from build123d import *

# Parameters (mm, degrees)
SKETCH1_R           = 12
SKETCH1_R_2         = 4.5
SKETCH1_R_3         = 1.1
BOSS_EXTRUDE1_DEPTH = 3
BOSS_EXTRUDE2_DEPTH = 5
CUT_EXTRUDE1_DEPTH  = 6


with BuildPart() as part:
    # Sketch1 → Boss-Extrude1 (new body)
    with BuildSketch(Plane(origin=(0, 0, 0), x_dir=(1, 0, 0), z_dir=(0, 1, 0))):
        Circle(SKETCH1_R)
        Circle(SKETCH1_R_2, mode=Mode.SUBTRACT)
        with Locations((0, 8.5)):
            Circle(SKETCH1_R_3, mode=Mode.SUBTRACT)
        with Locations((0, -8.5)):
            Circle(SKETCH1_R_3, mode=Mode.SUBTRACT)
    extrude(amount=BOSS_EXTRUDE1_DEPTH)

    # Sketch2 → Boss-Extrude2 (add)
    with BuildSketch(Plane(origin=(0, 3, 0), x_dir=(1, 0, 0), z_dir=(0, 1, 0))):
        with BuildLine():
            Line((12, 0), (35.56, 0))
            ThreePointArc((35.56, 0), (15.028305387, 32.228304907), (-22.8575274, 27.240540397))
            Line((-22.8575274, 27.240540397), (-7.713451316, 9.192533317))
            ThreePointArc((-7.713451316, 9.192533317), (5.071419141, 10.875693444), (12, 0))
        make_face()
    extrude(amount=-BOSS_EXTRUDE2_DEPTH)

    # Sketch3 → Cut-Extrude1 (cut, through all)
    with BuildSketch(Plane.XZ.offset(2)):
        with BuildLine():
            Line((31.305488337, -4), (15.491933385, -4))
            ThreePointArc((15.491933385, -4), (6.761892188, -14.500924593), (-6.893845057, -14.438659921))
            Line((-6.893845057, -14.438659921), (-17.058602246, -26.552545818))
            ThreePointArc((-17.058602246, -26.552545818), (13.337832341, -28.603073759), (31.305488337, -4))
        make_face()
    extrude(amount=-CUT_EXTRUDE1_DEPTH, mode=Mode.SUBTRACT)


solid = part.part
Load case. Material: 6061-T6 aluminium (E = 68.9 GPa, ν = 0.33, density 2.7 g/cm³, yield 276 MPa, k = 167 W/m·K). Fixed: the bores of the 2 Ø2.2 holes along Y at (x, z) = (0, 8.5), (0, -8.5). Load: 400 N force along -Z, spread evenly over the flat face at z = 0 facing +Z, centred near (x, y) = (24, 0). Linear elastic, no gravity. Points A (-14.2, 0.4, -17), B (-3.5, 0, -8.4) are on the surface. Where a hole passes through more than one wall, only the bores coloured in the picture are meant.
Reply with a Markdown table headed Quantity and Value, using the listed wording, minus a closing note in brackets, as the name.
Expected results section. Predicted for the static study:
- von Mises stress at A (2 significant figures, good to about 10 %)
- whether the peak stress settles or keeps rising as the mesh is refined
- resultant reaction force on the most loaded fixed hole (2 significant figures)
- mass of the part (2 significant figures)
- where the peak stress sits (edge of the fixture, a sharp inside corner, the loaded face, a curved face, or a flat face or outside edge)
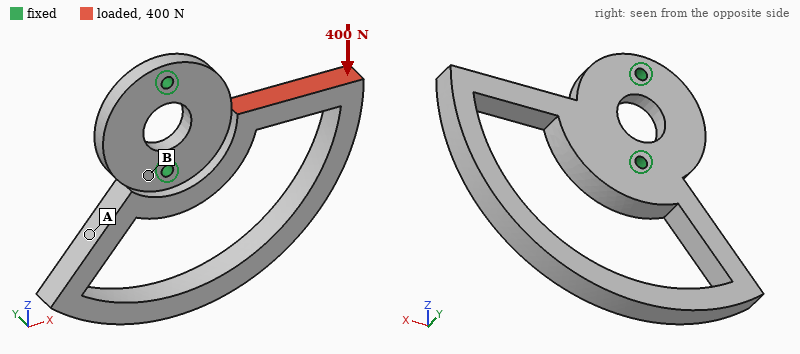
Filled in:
| Quantity | Value |
|---|---|
| von Mises stress at A | 39 MPa |
| whether the peak stress settles or keeps rising as the mesh is refined | keeps rising |
| resultant reaction force on the most loaded fixed hole | 570 N |
| mass of the part | 11 g |
| where the peak stress sits | a sharp inside corner |
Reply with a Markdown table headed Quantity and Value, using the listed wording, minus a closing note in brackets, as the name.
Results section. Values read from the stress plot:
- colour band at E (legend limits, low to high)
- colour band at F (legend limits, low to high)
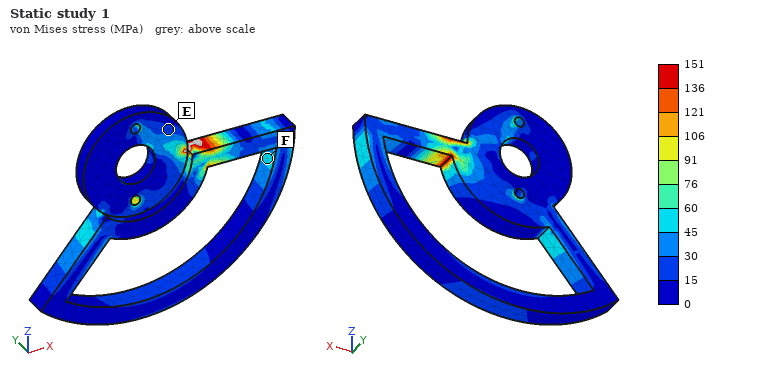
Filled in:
| Quantity | Value |
|---|---|
| colour band at E | 15 to 30 MPa |
| colour band at F | 45 to 60 MPa |
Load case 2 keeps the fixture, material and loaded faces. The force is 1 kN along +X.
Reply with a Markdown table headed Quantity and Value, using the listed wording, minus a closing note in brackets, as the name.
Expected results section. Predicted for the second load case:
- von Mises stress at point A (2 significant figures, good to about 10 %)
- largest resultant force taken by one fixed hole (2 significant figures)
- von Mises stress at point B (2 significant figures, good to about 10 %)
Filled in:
| Quantity | Value |
|---|---|
| von Mises stress at point A | 26 MPa |
| largest resultant force taken by one fixed hole | 580 N |
| von Mises stress at point B | 19 MPa |
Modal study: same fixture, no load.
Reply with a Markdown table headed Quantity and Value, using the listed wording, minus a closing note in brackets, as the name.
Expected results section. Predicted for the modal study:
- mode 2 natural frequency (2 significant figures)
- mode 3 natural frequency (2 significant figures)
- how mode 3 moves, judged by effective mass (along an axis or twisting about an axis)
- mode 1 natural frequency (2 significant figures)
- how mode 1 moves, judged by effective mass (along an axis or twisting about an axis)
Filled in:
| Quantity | Value |
|---|---|
| mode 2 natural frequency | 2200 Hz |
| mode 3 natural frequency | 2600 Hz |
| how mode 3 moves, judged by effective mass | along X |
| mode 1 natural frequency | 1400 Hz |
| how mode 1 moves, judged by effective mass | along Y |
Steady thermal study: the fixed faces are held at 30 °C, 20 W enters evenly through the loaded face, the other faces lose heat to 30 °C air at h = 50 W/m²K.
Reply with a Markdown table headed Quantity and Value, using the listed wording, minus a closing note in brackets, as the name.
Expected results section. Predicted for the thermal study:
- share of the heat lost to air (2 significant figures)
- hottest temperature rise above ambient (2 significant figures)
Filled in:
| Quantity | Value |
|---|---|
| share of the heat lost to air | 18 % |
| hottest temperature rise above ambient | 68 K |
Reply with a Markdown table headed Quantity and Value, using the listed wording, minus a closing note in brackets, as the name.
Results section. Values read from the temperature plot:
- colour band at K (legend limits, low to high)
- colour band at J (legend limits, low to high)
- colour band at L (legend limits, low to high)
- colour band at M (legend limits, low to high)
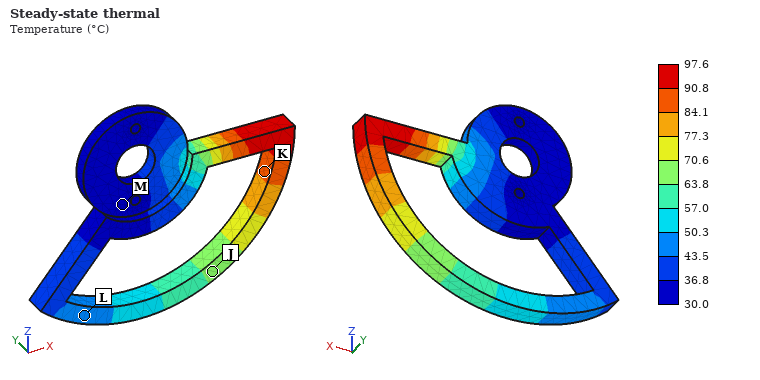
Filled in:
| Quantity | Value |
|---|---|
| colour band at K | 84.1 to 90.8 °C |
| colour band at J | 63.8 to 70.6 °C |
| colour band at L | 43.5 to 50.3 °C |
| colour band at M | 30.0 to 36.8 °C |
